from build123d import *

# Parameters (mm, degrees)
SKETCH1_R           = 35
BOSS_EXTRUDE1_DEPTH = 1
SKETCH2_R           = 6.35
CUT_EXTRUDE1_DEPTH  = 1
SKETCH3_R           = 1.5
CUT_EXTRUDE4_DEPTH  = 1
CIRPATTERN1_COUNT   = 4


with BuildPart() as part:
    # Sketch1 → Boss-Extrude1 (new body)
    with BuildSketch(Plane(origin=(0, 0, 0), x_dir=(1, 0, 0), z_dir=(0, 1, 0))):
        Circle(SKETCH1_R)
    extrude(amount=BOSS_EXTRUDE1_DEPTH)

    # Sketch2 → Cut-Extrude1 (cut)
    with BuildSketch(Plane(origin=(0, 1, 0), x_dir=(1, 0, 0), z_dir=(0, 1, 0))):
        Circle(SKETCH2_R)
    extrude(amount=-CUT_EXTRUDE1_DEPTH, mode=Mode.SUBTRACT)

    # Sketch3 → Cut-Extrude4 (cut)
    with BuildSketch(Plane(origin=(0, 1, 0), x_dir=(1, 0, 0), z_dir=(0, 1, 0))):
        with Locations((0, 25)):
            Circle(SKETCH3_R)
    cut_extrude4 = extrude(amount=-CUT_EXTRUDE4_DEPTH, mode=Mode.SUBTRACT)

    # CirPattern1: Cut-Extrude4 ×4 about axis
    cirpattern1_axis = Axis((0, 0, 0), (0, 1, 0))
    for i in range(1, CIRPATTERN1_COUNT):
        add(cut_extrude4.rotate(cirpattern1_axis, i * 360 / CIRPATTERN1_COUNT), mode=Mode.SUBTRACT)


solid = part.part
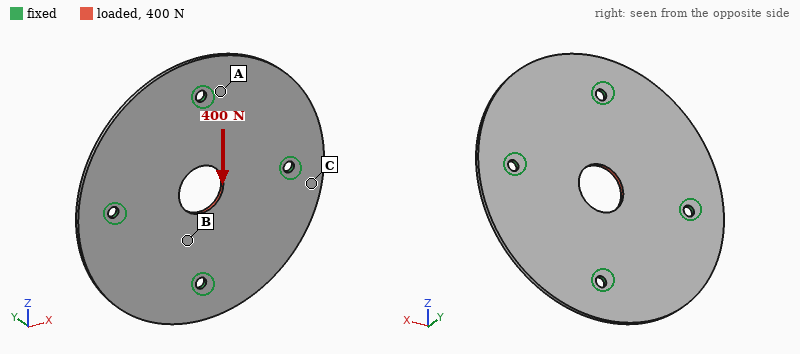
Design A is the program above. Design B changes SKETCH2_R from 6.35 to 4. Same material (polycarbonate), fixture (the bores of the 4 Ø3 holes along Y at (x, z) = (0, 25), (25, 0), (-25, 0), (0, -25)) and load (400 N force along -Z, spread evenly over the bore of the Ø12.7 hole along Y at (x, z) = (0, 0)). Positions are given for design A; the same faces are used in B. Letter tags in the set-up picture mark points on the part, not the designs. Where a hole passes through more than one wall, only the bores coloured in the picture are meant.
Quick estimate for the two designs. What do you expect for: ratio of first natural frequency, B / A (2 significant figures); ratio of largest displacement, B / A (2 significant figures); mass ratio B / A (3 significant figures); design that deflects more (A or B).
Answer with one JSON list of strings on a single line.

["1.0", "1.2", "1.02", "B"]
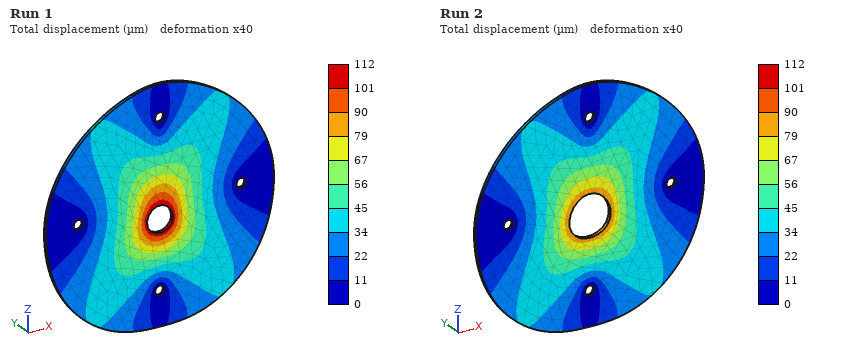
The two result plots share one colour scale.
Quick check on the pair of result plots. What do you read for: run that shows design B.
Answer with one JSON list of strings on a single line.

["Run 1"]
